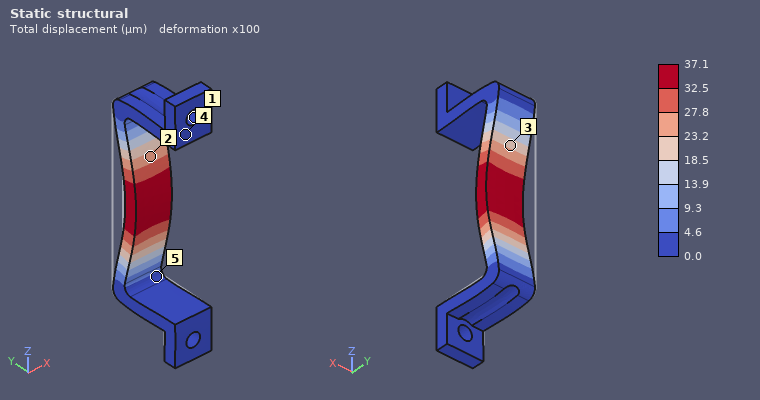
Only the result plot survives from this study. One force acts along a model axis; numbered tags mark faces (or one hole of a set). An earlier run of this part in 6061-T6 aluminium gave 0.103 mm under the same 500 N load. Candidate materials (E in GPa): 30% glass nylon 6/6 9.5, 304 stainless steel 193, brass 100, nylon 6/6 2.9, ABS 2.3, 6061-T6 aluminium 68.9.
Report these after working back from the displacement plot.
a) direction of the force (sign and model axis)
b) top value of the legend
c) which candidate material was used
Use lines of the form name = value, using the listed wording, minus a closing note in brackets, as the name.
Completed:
direction of the force = -Y
top value of the legend = 37.1 µm
which candidate material was used = 304 stainless steel
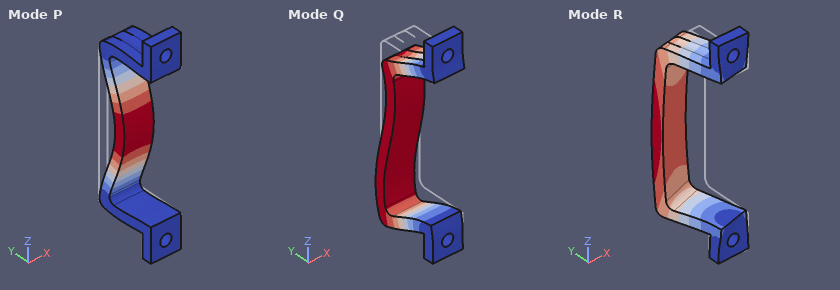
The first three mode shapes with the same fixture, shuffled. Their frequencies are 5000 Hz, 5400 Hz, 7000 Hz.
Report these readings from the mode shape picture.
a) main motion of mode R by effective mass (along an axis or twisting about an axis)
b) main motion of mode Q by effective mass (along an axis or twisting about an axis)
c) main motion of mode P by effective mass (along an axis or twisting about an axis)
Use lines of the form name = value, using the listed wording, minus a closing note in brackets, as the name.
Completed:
main motion of mode R by effective mass = along X
main motion of mode Q by effective mass = along Z
main motion of mode P by effective mass = along Y
